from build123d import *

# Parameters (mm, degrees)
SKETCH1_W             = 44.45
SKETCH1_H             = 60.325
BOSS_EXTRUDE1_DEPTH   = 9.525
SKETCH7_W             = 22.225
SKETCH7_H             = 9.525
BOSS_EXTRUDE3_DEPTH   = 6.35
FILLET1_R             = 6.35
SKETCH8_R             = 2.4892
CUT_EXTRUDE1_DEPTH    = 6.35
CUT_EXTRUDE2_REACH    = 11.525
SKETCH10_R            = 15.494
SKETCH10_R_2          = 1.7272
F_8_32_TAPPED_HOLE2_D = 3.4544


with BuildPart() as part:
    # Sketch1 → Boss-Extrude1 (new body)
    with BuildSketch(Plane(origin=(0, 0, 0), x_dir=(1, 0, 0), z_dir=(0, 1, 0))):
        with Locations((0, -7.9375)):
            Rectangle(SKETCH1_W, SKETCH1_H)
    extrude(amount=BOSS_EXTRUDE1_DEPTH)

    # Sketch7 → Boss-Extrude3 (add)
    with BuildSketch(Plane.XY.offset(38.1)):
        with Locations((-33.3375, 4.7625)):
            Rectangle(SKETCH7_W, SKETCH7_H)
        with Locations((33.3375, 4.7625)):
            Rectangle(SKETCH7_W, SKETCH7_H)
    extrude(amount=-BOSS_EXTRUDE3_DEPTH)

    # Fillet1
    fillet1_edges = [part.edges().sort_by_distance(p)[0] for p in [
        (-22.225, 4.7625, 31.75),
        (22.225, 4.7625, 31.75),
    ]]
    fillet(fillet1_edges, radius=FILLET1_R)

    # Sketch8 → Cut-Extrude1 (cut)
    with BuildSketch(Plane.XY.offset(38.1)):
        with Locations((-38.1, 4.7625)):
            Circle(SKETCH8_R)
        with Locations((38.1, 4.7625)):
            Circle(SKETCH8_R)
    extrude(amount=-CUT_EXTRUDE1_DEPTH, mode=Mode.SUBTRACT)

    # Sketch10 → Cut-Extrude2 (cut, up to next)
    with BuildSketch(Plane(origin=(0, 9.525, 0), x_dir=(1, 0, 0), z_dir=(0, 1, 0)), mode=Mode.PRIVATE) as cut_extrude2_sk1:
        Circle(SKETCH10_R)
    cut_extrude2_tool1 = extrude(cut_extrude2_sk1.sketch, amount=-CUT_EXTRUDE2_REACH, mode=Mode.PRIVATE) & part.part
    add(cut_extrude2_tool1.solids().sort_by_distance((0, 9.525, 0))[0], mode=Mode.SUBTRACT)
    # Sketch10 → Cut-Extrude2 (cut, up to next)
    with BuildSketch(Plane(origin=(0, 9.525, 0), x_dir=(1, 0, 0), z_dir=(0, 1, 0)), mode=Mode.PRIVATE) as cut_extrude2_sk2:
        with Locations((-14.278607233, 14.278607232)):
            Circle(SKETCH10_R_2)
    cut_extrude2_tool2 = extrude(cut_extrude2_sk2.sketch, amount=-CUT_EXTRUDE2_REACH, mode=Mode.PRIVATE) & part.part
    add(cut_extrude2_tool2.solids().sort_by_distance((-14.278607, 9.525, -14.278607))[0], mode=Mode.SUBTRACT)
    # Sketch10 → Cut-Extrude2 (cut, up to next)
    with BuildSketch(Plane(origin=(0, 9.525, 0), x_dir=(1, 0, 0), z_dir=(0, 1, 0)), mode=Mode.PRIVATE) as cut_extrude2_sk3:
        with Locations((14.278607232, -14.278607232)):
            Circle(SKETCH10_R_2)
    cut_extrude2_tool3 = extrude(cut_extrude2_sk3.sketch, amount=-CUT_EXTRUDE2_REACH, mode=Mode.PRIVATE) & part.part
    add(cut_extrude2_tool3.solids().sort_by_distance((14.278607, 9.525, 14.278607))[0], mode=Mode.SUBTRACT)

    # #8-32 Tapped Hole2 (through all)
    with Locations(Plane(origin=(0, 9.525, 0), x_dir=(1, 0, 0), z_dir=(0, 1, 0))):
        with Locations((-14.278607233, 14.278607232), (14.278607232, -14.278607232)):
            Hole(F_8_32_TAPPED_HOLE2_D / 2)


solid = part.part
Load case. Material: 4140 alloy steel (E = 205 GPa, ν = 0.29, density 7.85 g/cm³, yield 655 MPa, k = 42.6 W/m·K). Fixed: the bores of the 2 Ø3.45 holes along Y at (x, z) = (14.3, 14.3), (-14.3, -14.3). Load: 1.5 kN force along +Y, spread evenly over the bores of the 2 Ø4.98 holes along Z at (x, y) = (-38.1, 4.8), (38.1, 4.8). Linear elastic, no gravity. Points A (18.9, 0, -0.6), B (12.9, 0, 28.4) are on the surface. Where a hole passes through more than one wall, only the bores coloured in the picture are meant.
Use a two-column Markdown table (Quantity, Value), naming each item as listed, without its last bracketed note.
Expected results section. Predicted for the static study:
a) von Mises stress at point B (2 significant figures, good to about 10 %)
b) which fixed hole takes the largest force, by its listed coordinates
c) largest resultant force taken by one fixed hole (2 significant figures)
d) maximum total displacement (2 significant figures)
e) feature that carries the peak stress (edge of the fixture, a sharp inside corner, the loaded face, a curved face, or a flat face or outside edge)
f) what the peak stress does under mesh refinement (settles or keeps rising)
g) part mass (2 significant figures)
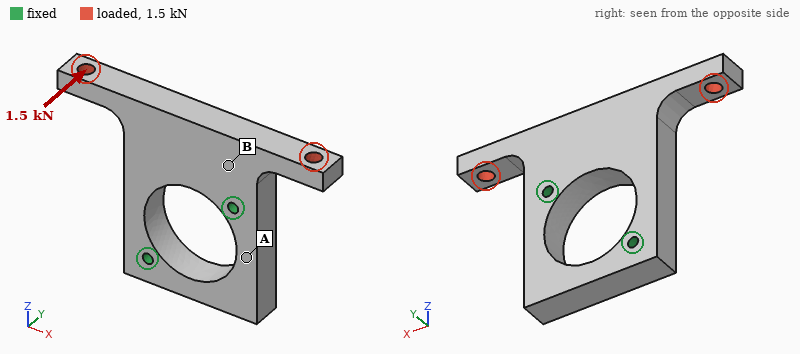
| Quantity | Value |
|---|---|
| von Mises stress at point B | 54 MPa |
| which fixed hole takes the largest force, by its listed coordinates | (14.3, 14.3) |
| largest resultant force taken by one fixed hole | 1.3 kN |
| maximum total displacement | 0.15 mm |
| feature that carries the peak stress | edge of the fixture |
| what the peak stress does under mesh refinement | keeps rising |
| part mass | 160 g |
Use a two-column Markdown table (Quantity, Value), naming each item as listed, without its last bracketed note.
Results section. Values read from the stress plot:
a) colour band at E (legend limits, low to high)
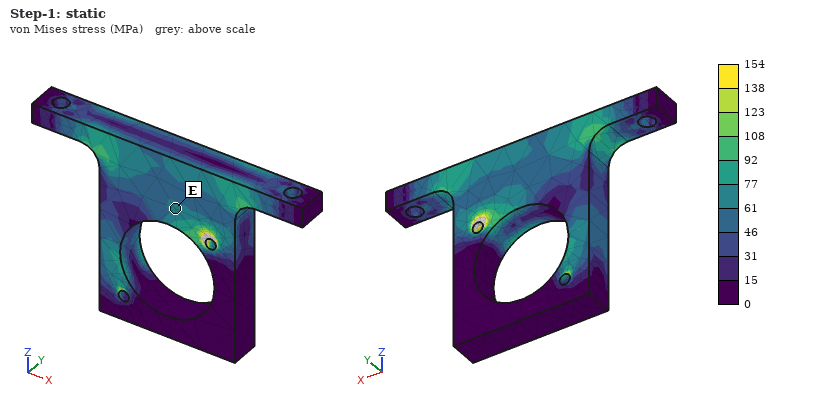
| Quantity | Value |
|---|---|
| colour band at E | 61 to 77 MPa |
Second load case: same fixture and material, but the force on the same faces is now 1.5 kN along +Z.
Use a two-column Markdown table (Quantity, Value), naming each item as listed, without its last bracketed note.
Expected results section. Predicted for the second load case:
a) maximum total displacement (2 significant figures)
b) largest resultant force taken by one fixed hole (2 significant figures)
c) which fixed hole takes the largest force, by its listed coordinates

| Quantity | Value |
|---|---|
| maximum total displacement | 52 µm |
| largest resultant force taken by one fixed hole | 860 N |
| which fixed hole takes the largest force, by its listed coordinates | (14.3, 14.3) |
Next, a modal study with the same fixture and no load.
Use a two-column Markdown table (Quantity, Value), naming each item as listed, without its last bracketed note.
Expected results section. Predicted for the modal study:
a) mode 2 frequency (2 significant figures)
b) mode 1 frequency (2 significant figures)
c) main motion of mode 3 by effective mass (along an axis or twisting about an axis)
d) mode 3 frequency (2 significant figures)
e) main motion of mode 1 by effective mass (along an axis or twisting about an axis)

| Quantity | Value |
|---|---|
| mode 2 frequency | 6700 Hz |
| mode 1 frequency | 3200 Hz |
| main motion of mode 3 by effective mass | along Y |
| mode 3 frequency | 7700 Hz |
| main motion of mode 1 by effective mass | along Y |
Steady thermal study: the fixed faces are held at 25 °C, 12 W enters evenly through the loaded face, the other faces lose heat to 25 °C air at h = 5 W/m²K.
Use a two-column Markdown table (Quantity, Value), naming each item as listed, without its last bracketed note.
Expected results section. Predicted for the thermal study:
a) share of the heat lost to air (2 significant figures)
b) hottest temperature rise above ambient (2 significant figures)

| Quantity | Value |
|---|---|
| share of the heat lost to air | 6.1 % |
| hottest temperature rise above ambient | 76 K |
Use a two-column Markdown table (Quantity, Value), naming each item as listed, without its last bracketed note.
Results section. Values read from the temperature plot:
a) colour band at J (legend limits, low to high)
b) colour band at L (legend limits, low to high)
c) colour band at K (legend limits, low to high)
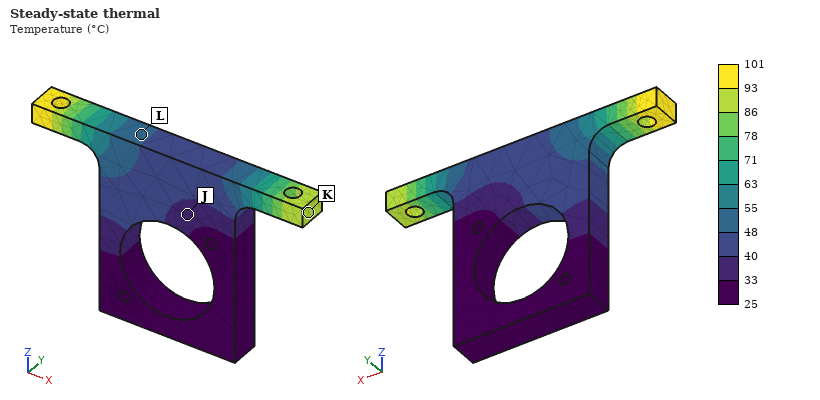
| Quantity | Value |
|---|---|
| colour band at J | 33 to 40 °C |
| colour band at L | 48 to 55 °C |
| colour band at K | 86 to 93 °C |
